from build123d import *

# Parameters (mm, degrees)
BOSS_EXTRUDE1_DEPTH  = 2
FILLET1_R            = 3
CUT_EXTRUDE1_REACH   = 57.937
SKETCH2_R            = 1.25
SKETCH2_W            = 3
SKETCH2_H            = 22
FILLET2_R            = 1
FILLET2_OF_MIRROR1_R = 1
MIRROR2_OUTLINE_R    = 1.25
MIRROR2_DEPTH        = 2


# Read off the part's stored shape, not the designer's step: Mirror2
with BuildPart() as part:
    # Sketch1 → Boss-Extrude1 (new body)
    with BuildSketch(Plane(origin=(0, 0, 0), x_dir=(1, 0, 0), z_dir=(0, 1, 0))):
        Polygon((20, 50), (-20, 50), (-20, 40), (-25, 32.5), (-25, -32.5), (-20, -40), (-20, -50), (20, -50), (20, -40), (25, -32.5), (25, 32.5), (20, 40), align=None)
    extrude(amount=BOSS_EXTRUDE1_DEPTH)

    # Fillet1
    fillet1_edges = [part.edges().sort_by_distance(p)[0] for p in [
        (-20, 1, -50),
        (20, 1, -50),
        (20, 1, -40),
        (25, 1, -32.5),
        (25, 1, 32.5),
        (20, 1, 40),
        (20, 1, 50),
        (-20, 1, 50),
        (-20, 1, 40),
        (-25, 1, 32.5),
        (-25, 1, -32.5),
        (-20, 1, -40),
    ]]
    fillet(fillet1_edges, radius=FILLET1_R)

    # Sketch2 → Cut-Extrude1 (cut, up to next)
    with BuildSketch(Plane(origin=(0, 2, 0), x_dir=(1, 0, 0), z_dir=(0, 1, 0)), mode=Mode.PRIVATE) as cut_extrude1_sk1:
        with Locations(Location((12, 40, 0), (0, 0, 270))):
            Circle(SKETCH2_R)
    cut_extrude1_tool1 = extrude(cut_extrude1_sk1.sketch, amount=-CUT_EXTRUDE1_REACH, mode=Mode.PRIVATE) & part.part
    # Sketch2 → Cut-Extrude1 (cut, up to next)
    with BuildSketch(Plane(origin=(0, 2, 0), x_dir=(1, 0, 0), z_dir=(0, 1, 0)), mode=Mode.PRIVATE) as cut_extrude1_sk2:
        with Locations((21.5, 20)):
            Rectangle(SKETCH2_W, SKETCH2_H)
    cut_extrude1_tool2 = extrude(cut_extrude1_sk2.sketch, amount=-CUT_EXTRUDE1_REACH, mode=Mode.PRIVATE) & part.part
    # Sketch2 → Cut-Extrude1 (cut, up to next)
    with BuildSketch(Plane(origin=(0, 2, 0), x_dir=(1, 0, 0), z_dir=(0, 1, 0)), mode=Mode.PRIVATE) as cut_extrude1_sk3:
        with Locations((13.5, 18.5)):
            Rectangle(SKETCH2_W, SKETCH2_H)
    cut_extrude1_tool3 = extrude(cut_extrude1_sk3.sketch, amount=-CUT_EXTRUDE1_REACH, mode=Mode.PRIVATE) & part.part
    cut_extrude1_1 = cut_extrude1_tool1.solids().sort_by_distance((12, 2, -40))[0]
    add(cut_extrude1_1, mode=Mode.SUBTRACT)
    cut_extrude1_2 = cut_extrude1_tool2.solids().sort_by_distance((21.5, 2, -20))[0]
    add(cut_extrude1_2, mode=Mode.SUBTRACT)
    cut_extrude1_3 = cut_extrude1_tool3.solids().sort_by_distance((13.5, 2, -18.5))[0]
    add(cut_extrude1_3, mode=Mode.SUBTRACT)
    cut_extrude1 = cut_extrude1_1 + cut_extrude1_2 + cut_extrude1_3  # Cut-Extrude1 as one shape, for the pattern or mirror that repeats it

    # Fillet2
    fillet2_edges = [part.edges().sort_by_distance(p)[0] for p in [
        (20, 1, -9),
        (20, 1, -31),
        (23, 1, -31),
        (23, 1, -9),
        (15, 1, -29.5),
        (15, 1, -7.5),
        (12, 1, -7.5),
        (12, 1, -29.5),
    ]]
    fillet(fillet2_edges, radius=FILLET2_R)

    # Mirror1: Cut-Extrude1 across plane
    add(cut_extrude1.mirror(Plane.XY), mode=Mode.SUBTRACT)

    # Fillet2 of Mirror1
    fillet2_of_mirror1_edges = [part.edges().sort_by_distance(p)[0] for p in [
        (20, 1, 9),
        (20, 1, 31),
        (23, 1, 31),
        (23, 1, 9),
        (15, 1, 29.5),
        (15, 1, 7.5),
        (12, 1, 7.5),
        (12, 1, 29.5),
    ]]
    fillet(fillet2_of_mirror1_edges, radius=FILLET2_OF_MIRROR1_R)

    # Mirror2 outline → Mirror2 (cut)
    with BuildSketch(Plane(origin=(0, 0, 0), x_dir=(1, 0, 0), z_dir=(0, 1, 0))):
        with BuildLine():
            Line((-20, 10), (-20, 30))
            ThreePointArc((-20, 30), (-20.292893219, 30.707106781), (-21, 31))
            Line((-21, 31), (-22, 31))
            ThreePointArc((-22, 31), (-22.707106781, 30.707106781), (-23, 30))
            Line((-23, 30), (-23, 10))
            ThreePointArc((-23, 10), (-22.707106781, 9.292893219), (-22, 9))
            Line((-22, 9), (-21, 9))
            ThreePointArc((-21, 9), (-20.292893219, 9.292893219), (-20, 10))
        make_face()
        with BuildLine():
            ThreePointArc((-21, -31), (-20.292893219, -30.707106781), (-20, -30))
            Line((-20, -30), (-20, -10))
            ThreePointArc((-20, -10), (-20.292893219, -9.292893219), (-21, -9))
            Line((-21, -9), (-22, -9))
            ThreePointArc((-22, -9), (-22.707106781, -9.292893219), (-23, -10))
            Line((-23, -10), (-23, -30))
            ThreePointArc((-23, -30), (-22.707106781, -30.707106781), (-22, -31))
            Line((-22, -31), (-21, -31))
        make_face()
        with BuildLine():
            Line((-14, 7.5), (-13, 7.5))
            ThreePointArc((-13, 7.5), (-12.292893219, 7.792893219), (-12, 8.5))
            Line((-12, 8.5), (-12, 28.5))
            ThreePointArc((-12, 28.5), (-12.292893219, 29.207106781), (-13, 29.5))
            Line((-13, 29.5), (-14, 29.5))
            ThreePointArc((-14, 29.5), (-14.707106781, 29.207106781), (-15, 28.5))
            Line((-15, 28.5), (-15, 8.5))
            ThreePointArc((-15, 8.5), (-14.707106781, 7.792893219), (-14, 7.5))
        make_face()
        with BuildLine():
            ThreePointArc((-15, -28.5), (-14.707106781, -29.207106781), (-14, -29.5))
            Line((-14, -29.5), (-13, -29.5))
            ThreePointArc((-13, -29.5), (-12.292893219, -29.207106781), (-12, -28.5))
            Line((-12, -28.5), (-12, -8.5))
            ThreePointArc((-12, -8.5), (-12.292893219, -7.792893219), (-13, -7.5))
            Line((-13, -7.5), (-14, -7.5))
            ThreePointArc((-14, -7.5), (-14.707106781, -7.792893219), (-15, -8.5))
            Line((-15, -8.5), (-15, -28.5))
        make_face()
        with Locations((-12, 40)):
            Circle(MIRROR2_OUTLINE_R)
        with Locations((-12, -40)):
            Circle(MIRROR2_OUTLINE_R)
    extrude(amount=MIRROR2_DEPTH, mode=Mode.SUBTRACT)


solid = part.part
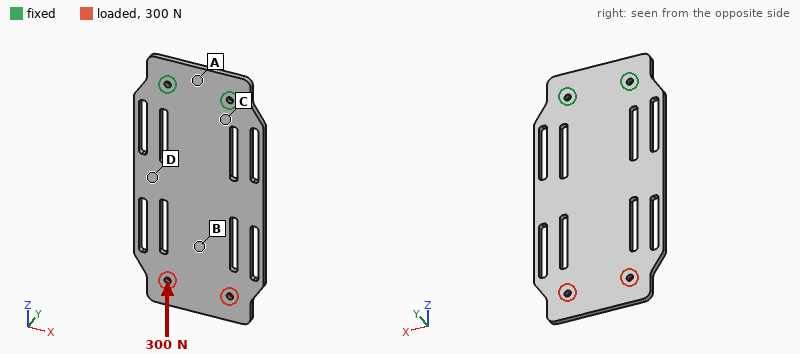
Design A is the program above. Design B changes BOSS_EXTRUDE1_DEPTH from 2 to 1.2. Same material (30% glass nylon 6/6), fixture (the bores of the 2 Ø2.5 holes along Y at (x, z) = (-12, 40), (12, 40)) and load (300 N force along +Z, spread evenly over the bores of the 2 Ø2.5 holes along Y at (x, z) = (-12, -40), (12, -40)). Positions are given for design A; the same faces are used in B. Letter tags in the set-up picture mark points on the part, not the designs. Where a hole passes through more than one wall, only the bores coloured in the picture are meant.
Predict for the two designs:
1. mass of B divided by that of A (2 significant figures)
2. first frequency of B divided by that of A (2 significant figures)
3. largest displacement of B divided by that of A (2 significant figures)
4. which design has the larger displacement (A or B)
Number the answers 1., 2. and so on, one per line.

1. 0.60
2. 0.61
3. 1.7
4. B
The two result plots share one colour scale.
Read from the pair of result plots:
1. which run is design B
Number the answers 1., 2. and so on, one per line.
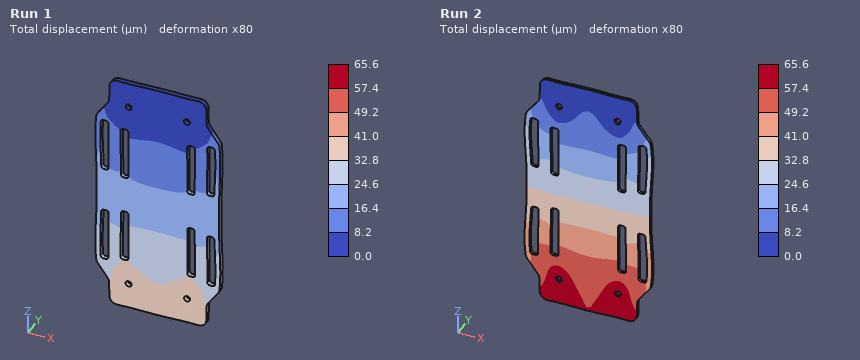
1. Run 2
